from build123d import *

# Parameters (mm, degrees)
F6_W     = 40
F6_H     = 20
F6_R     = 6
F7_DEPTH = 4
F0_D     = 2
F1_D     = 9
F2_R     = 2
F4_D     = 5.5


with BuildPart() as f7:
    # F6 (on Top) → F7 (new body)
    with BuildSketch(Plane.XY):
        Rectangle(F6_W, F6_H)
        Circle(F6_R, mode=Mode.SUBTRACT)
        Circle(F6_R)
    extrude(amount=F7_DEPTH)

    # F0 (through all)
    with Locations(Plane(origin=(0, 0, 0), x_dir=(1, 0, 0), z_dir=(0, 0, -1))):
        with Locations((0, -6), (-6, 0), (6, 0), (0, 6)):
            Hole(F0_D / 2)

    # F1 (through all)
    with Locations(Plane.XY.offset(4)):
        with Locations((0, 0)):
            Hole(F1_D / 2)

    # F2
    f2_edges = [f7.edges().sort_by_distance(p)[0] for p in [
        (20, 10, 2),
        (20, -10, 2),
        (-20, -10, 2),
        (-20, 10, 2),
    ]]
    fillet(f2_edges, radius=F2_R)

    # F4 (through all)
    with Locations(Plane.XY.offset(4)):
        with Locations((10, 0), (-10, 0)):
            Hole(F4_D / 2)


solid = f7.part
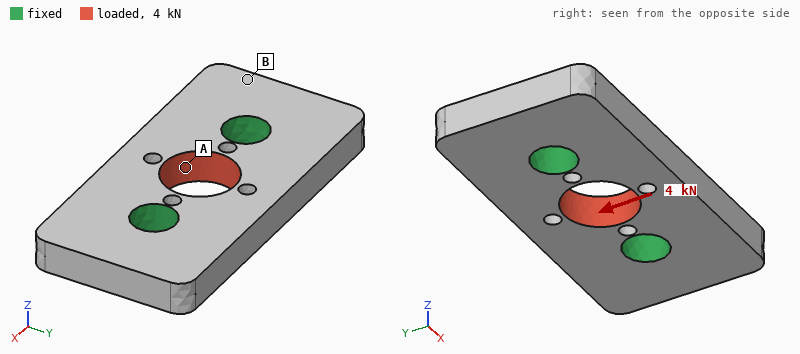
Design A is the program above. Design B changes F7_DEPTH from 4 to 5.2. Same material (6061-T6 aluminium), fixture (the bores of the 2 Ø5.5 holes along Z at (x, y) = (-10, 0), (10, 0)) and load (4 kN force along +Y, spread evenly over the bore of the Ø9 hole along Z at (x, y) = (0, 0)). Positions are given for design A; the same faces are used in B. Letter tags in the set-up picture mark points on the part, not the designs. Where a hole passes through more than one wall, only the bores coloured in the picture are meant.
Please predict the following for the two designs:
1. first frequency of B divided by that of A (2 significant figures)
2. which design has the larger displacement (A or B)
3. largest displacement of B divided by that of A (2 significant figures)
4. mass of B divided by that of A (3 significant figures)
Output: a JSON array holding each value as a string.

["1.2", "A", "0.77", "1.30"]
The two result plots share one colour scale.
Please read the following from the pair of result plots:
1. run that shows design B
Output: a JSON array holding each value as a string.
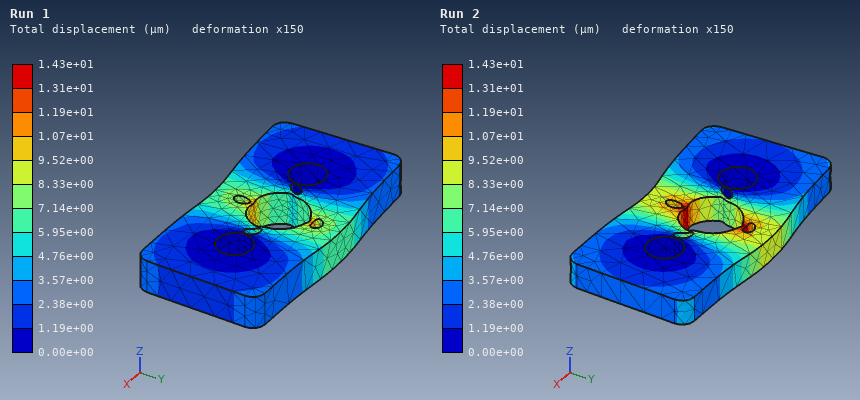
["Run 1"]
